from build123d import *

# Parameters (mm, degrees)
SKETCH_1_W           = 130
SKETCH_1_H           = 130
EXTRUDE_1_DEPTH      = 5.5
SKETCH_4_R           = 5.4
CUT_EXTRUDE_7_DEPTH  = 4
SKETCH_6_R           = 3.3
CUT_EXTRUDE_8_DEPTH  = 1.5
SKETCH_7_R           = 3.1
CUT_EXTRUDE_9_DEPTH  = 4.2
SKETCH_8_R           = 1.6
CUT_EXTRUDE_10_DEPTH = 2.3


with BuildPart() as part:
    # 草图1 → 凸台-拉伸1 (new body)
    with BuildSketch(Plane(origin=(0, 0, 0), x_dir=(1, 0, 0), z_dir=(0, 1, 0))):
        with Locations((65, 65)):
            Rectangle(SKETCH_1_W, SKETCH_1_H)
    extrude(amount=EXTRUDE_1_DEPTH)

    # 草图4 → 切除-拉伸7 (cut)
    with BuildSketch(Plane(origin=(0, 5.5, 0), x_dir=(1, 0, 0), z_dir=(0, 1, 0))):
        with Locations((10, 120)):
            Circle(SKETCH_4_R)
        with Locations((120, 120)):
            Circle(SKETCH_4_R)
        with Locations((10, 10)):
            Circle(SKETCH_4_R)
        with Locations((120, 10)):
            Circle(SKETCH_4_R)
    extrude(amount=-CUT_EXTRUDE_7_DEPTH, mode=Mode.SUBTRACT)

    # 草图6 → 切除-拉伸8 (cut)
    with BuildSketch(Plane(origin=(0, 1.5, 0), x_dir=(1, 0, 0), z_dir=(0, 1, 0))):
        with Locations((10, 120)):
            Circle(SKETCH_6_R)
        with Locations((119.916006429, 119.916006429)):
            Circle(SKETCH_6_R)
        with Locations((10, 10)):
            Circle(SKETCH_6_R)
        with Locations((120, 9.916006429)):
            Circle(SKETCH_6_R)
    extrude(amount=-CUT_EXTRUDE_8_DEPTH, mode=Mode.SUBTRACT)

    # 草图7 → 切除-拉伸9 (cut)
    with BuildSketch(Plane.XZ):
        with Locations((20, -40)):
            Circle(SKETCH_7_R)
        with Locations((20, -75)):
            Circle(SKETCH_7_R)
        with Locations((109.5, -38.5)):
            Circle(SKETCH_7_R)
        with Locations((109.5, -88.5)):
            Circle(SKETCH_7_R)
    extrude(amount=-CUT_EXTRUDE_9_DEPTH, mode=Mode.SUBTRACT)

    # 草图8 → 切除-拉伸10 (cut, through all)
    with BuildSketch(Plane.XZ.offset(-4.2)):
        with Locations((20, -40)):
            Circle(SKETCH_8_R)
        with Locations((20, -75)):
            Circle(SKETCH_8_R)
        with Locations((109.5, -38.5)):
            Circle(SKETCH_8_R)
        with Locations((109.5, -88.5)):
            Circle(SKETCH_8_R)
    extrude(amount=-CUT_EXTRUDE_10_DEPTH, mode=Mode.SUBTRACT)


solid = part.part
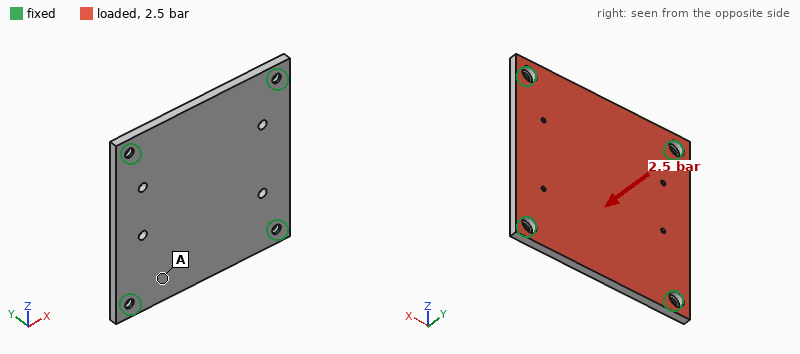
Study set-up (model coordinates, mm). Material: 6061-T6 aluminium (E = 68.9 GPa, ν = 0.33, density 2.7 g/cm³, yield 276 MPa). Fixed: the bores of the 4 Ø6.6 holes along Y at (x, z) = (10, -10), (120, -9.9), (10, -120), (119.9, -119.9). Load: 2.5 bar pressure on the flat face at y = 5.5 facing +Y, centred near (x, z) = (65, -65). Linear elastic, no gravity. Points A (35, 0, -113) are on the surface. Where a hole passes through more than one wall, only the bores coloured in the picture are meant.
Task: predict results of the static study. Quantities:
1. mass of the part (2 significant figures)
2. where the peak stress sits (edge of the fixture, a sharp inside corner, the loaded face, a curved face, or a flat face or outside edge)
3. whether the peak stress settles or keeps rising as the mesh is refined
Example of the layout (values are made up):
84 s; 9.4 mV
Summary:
240 g; edge of the fixture; keeps rising
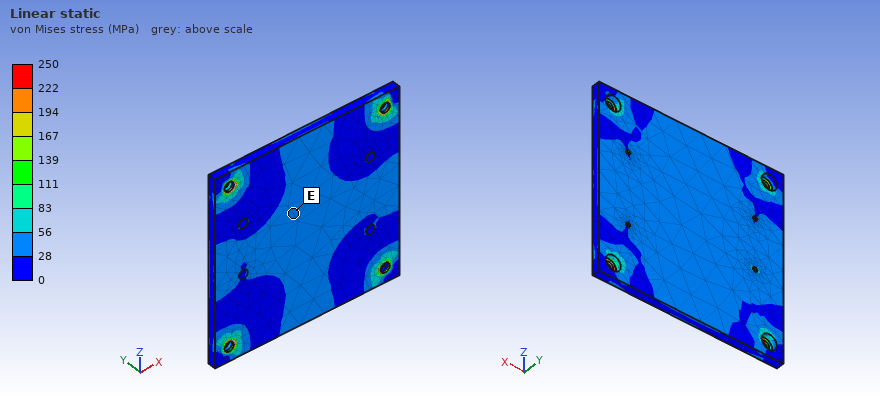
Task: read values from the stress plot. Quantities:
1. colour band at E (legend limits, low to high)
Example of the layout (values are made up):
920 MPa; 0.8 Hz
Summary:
28 to 56 MPa
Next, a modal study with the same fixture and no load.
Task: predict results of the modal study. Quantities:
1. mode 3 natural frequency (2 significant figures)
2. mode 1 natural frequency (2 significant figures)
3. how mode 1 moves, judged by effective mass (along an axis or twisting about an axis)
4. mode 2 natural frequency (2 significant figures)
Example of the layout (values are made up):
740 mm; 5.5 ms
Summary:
2200 Hz; 1300 Hz; along Y; 2200 Hz
